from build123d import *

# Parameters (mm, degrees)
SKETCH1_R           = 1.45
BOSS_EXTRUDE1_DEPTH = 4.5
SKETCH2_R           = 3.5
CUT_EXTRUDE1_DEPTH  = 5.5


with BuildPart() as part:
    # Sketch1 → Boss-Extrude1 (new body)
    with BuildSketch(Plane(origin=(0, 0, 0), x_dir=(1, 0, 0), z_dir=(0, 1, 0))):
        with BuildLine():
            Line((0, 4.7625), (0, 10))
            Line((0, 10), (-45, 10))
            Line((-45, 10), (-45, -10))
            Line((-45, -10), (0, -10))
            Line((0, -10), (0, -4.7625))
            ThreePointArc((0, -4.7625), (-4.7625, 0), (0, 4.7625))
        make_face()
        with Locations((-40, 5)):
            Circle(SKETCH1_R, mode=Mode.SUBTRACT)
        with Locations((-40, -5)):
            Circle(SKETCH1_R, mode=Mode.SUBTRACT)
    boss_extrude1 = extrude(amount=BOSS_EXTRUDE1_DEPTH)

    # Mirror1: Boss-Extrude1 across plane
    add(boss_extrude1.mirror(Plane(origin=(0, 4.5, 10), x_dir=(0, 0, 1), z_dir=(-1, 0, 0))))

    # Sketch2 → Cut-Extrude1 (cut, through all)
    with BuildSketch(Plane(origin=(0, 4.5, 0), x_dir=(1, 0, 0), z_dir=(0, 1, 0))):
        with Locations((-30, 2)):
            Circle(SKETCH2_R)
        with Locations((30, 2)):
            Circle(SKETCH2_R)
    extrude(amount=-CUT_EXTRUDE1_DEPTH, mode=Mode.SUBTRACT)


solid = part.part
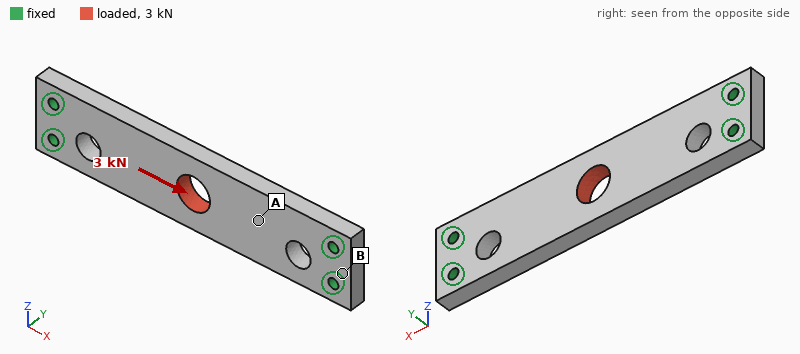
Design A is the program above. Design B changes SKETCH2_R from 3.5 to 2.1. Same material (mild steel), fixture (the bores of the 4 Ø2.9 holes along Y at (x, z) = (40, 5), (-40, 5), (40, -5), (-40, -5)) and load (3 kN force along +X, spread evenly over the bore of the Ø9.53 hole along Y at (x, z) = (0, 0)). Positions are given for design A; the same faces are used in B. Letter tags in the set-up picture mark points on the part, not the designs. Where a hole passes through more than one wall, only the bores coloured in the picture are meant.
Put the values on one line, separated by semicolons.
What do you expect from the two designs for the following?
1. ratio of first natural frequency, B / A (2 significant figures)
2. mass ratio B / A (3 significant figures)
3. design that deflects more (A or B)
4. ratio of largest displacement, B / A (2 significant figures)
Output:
1.0; 1.03; A; 0.90
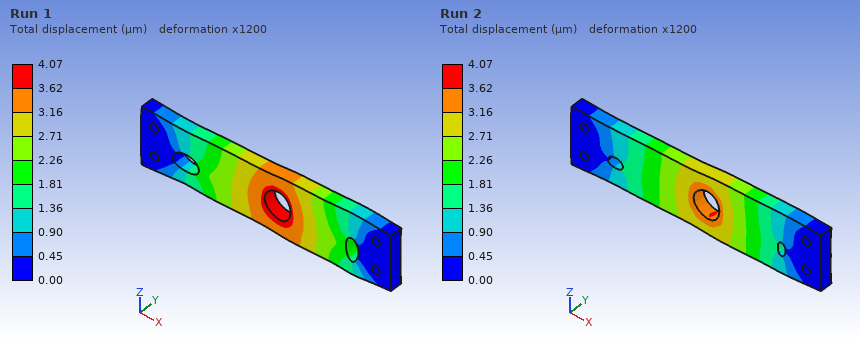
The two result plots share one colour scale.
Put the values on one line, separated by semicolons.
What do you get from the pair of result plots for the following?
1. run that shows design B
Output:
Run 2
